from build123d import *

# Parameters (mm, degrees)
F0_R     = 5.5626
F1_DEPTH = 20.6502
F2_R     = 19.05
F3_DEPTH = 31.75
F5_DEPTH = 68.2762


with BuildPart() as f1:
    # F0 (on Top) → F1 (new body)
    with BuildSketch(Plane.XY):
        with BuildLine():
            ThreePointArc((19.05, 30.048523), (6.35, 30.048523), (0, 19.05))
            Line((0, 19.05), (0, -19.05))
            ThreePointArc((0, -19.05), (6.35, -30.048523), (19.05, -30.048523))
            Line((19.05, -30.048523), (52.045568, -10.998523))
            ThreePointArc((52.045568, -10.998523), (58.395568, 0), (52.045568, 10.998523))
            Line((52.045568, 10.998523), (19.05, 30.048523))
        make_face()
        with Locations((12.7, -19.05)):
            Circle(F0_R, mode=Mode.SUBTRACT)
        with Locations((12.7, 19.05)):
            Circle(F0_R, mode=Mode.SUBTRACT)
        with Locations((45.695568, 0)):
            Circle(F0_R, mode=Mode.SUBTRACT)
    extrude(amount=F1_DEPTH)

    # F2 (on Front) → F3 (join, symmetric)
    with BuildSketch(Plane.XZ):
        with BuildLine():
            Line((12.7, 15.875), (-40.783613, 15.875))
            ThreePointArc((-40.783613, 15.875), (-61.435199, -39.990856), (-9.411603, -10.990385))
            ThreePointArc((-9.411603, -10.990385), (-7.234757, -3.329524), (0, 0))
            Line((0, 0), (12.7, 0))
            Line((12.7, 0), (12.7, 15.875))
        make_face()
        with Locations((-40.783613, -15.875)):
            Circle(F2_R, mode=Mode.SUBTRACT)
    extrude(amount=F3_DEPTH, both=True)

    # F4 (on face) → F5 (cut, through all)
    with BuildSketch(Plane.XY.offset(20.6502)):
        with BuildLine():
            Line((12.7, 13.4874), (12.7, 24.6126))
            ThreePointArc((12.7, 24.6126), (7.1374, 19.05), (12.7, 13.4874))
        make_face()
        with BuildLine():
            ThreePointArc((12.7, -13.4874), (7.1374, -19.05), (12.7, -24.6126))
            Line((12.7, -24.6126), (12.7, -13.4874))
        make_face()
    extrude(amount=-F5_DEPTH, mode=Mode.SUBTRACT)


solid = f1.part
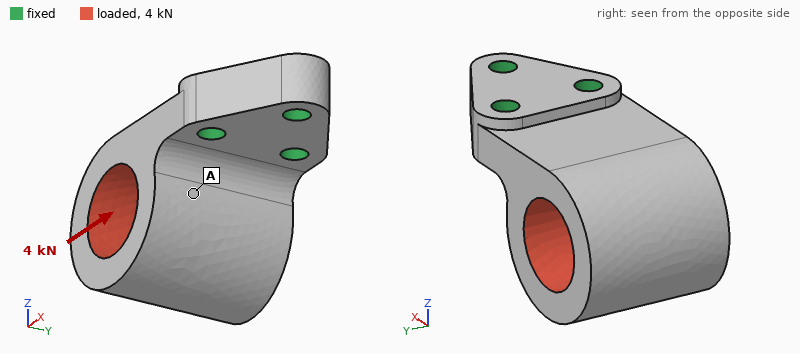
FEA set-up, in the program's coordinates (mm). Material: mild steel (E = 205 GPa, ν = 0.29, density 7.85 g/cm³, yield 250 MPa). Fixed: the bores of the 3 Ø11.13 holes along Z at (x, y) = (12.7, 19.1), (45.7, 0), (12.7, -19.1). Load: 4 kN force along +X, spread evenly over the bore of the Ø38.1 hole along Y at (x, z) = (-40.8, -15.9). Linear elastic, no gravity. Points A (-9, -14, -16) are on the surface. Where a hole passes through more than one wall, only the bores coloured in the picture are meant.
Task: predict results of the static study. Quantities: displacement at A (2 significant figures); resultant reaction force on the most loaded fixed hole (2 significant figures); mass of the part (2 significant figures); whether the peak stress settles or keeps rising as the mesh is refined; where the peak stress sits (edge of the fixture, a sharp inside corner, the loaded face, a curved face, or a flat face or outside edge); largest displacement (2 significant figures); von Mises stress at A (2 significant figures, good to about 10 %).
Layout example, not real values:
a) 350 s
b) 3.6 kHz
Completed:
a) 12 µm
b) 1.9 kN
c) 1.6 kg
d) keeps rising
e) edge of the fixture
f) 39 µm
g) 7.7 MPa
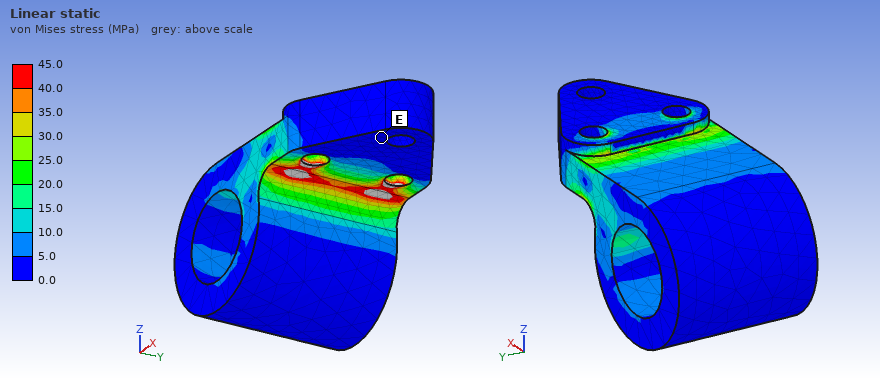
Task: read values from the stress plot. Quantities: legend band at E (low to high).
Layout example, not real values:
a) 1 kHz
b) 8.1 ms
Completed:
a) 0.0 to 5.0 MPa
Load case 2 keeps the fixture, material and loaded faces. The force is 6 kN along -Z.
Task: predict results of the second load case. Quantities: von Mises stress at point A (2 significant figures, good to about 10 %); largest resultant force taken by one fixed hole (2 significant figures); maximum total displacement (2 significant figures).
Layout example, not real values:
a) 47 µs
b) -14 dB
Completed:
a) 10 MPa
b) 3.5 kN
c) 95 µm
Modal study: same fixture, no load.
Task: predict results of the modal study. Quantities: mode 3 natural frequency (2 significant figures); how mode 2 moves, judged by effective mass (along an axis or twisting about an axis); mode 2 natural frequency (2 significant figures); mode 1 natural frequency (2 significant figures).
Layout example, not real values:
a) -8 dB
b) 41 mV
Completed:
a) 5100 Hz
b) along Y
c) 3100 Hz
d) 1300 Hz
